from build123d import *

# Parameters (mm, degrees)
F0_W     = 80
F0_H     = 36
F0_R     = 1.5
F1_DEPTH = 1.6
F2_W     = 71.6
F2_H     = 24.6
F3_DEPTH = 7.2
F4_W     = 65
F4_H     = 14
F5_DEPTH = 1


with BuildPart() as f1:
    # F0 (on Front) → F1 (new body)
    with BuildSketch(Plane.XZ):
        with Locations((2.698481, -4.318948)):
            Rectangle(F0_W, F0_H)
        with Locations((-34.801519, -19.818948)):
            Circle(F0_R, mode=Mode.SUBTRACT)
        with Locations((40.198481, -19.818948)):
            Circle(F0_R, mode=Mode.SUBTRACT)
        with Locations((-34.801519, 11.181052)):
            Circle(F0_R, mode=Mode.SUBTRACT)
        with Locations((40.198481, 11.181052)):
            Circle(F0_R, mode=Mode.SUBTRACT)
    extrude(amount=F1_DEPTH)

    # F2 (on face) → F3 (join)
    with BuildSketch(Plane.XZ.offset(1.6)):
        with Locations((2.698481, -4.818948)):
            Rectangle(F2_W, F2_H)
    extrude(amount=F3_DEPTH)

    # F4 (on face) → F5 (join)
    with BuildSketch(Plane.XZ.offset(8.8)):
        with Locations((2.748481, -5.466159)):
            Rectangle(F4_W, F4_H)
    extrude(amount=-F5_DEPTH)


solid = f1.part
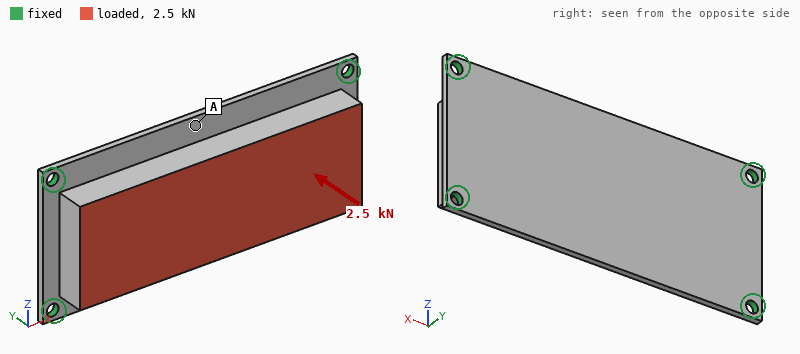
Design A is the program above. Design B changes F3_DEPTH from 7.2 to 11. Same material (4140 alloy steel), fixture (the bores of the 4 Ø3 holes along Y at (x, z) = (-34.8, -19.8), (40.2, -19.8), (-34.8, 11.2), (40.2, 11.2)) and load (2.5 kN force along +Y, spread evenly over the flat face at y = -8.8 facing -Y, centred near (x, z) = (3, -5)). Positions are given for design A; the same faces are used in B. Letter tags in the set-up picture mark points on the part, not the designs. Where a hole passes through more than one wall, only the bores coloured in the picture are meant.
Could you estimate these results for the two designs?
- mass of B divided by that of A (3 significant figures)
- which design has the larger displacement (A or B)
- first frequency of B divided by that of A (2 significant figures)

1.39
A
1.1
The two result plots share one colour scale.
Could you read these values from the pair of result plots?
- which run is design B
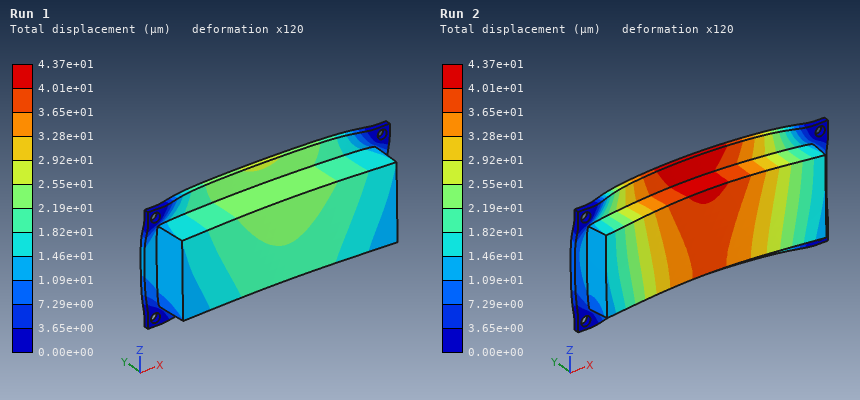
Run 1
